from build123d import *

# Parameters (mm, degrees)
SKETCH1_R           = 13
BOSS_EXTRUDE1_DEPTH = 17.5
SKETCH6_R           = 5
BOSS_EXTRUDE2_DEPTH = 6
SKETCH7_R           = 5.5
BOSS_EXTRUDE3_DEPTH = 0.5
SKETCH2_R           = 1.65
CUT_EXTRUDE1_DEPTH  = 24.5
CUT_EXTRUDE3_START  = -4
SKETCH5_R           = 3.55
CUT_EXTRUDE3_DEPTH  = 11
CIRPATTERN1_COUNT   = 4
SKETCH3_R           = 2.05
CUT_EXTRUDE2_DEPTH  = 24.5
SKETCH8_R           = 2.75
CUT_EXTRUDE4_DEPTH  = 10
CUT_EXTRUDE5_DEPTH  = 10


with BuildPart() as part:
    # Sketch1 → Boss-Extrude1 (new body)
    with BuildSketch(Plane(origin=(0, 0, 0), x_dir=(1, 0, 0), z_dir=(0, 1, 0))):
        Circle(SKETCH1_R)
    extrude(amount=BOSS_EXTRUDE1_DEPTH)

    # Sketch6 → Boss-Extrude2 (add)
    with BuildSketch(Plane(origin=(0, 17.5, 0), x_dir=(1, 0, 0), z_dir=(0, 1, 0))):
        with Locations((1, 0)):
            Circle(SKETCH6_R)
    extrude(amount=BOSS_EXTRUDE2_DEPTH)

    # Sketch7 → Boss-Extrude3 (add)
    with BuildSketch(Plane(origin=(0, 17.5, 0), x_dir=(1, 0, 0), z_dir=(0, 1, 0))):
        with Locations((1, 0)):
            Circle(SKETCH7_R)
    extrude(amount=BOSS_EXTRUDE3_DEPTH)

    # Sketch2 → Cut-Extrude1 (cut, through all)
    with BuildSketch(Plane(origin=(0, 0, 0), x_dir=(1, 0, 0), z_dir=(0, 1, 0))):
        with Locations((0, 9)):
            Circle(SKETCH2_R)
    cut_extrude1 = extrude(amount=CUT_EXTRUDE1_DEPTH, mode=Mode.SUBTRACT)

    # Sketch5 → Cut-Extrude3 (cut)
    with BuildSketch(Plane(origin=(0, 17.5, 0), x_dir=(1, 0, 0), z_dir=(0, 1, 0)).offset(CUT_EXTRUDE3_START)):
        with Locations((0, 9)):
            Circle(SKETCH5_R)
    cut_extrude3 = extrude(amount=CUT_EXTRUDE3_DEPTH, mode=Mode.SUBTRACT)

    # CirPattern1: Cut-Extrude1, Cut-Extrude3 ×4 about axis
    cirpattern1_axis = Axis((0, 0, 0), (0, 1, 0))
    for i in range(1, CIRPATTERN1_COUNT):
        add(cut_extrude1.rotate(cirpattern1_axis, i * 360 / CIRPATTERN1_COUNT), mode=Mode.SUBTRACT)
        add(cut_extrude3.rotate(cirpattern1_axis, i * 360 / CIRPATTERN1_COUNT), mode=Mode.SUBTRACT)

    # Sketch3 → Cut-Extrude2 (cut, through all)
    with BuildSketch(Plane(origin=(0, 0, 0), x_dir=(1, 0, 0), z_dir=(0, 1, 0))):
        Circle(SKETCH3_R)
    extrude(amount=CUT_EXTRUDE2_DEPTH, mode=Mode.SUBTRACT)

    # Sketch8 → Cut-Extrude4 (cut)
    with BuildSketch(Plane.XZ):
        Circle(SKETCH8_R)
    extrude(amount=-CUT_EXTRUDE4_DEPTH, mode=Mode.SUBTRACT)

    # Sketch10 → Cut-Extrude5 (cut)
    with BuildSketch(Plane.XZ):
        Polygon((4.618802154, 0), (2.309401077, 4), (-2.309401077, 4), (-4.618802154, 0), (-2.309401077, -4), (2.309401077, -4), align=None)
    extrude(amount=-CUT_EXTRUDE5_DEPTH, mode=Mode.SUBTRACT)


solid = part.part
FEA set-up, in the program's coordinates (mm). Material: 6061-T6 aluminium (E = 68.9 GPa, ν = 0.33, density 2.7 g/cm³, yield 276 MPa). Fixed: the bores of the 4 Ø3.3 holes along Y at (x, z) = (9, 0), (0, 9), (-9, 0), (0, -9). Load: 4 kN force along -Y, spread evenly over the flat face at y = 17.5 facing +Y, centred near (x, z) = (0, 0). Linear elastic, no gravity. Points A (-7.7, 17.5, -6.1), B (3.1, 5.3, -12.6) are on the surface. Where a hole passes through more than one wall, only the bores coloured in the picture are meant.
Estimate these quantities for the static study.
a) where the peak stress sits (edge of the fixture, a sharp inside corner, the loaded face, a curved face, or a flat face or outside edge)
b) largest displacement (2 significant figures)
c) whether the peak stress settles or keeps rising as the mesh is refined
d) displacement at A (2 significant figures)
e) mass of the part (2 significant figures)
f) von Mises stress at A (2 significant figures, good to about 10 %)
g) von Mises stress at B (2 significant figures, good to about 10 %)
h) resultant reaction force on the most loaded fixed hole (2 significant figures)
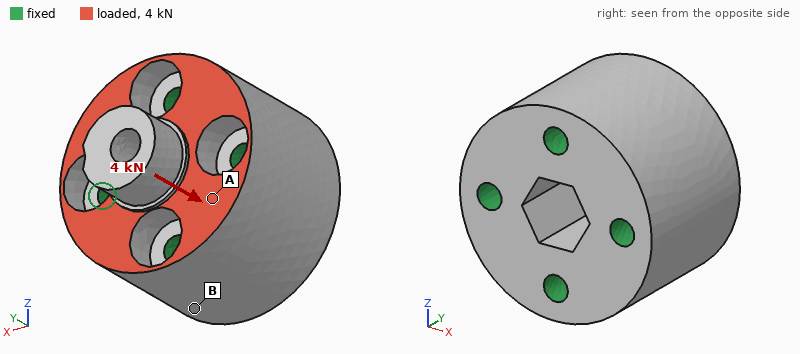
edge of the fixture
2.8 µm
keeps rising
2.3 µm
21 g
14 MPa
4.7 MPa
1.1 kN
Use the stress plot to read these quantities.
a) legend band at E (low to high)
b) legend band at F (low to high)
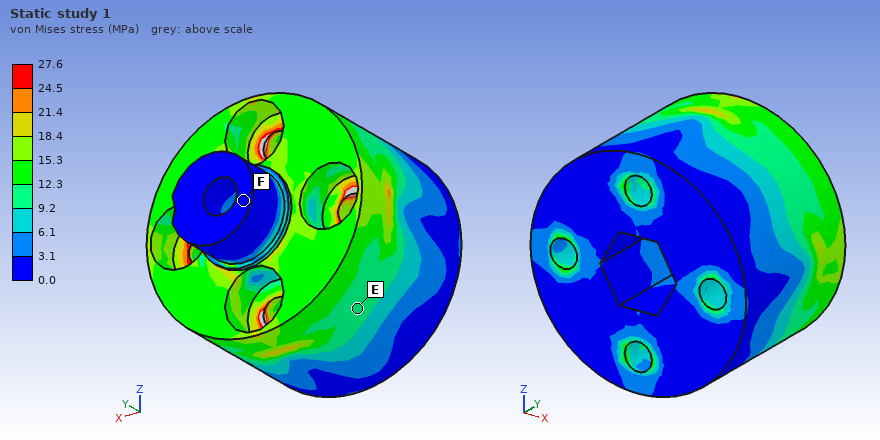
9.2 to 12.3 MPa
0.0 to 3.1 MPa
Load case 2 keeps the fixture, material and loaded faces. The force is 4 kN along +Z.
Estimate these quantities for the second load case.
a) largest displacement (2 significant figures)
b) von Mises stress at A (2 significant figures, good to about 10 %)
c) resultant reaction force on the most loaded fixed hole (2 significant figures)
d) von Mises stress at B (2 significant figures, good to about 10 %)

11 µm
33 MPa
1.4 kN
7.9 MPa
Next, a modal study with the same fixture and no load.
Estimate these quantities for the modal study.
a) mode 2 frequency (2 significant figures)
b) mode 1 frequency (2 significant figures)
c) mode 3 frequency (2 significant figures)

56 kHz
56 kHz
81 kHz
